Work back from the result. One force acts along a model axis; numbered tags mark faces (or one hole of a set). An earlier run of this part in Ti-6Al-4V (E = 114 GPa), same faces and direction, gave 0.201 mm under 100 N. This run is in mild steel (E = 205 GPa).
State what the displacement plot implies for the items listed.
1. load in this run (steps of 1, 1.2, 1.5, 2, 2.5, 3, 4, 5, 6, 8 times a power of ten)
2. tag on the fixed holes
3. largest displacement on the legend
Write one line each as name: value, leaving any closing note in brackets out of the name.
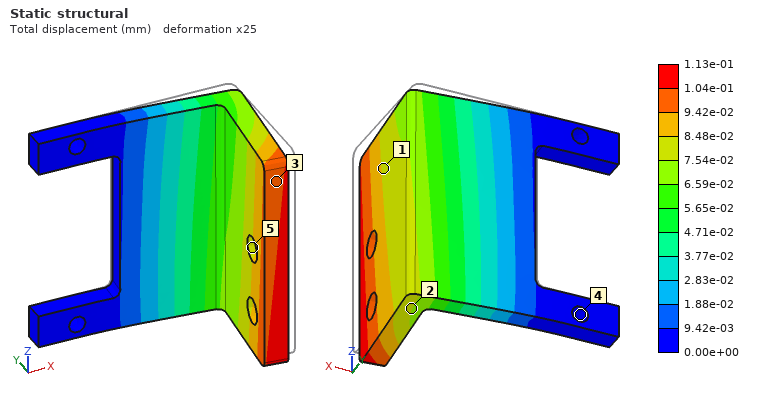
load in this run: 100 N
tag on the fixed holes: 4
largest displacement on the legend: 1.13e-01 mm
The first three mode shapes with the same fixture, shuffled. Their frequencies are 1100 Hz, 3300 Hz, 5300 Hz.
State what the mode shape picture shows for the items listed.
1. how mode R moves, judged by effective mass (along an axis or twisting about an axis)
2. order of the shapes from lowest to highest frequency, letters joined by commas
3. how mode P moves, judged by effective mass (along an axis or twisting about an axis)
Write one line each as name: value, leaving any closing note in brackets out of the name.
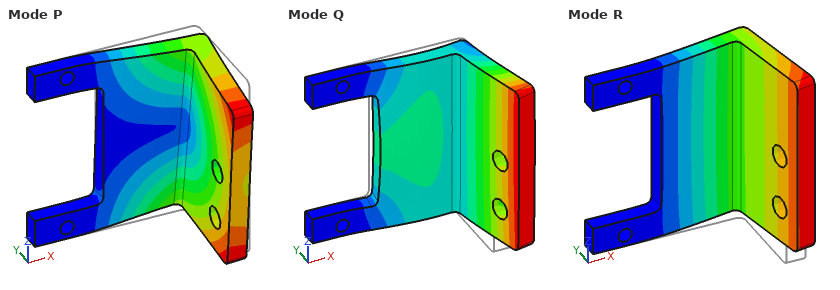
how mode R moves, judged by effective mass: along Y
order of the shapes from lowest to highest frequency, letters joined by commas: R, P, Q
how mode P moves, judged by effective mass: along Z
